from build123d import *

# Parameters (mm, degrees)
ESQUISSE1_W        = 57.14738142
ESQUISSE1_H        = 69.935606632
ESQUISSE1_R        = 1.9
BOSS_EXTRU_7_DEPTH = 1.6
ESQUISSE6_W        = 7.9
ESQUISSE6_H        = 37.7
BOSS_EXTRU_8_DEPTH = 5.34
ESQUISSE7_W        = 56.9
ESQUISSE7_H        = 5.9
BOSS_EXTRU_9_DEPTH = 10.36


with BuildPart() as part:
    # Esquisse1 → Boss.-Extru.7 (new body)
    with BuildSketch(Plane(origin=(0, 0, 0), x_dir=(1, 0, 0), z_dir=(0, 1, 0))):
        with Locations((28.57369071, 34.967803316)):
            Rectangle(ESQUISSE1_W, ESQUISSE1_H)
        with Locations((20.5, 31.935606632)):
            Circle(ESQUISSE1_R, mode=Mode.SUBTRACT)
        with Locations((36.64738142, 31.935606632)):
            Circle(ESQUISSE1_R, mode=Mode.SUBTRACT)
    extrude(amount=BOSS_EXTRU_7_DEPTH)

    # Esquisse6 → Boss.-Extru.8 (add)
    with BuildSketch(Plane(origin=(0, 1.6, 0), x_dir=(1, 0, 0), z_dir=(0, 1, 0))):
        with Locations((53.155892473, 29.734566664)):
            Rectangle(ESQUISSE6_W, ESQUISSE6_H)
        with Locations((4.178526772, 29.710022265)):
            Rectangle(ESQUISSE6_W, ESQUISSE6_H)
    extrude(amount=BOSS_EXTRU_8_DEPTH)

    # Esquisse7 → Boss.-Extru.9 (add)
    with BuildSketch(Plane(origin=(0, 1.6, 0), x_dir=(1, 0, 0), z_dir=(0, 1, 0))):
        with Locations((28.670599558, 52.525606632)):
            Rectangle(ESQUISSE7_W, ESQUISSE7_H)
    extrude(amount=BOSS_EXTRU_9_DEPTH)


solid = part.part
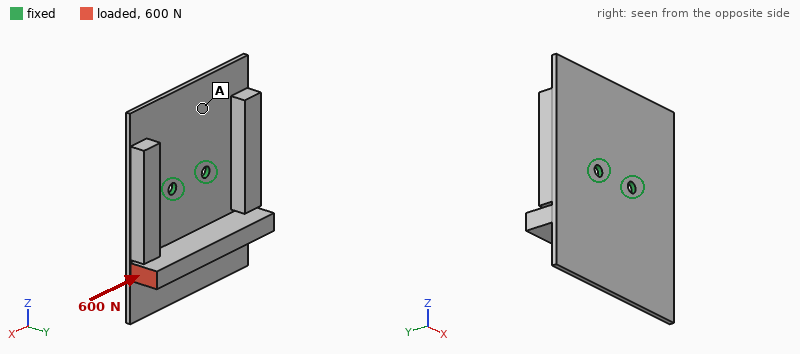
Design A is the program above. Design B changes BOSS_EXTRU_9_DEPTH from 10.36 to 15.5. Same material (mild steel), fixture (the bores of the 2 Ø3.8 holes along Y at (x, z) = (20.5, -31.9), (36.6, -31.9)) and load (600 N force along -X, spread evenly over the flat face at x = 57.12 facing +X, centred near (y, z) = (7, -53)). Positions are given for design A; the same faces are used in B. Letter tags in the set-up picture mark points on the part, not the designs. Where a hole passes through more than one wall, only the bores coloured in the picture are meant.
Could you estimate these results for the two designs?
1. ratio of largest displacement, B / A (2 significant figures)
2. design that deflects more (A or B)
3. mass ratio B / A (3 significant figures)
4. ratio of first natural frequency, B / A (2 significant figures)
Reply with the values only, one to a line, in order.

1.5
B
1.13
0.89
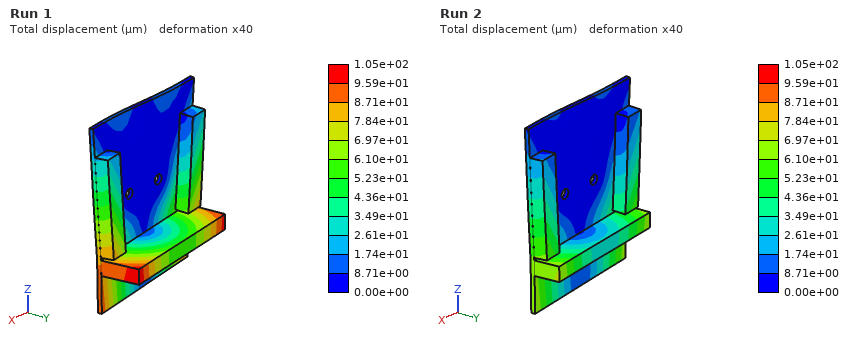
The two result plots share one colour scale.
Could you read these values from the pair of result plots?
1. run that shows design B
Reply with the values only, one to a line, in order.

Run 1
